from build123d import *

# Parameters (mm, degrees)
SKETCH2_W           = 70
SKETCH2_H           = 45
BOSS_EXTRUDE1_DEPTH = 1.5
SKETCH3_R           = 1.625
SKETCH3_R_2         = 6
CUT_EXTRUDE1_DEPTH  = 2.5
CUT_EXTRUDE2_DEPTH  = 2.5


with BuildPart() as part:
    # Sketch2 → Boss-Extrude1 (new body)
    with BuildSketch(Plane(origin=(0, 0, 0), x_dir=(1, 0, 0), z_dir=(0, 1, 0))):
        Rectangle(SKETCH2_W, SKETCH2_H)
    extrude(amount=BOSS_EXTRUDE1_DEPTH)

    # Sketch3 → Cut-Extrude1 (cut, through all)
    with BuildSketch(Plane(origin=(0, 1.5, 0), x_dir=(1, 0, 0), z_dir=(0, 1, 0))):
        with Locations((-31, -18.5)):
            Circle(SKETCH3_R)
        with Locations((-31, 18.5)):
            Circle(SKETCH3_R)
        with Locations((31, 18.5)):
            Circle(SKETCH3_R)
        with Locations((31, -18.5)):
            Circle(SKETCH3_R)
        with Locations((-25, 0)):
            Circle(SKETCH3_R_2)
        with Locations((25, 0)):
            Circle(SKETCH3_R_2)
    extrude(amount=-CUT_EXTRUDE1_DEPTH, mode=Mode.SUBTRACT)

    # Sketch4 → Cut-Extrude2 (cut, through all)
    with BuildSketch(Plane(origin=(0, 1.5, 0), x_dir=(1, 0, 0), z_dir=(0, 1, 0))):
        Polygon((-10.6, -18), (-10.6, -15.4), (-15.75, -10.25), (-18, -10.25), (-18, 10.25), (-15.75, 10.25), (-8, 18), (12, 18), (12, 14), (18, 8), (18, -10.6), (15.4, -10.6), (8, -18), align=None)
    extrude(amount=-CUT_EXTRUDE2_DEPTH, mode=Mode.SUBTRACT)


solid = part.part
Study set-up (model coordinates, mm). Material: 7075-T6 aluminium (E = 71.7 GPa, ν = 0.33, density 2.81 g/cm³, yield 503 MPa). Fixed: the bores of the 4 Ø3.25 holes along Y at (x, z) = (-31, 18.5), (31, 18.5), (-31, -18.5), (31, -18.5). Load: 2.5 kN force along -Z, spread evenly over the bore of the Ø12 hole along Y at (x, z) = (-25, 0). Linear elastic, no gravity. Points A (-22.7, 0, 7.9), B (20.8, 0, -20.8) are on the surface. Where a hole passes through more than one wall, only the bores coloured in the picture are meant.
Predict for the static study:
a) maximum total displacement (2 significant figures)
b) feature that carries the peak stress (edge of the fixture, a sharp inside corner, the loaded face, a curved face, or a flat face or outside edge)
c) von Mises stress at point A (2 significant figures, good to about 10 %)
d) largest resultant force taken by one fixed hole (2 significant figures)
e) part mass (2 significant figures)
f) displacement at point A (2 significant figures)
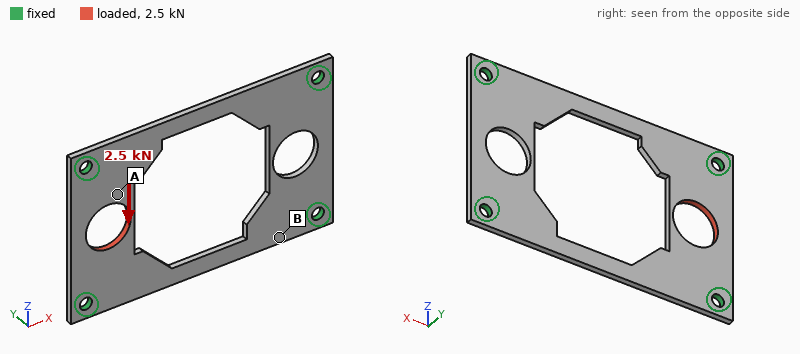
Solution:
44 µm
edge of the fixture
66 MPa
1.2 kN
7.5 g
29 µm
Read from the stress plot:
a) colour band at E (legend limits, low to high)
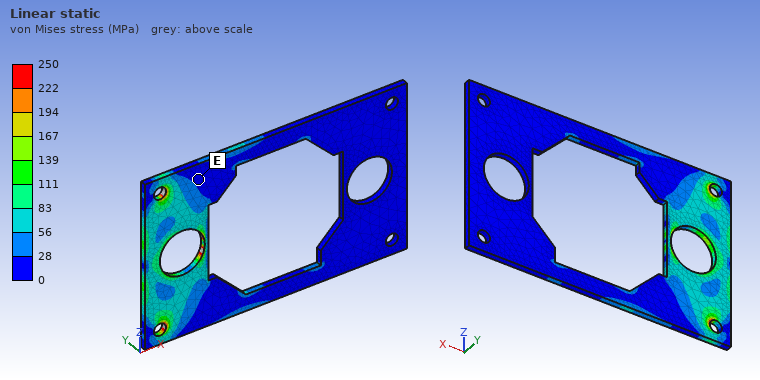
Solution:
0 to 28 MPa
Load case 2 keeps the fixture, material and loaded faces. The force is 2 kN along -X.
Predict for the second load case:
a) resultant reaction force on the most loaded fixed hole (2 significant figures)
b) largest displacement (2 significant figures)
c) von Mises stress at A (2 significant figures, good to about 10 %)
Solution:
1.1 kN
69 µm
110 MPa
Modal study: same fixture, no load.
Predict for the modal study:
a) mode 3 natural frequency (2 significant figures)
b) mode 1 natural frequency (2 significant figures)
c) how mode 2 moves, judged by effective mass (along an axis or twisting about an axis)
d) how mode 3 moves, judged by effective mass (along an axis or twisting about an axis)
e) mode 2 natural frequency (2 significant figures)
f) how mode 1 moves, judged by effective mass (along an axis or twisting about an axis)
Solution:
4800 Hz
2600 Hz
twisting about X
twisting about Z
2800 Hz
along Y
